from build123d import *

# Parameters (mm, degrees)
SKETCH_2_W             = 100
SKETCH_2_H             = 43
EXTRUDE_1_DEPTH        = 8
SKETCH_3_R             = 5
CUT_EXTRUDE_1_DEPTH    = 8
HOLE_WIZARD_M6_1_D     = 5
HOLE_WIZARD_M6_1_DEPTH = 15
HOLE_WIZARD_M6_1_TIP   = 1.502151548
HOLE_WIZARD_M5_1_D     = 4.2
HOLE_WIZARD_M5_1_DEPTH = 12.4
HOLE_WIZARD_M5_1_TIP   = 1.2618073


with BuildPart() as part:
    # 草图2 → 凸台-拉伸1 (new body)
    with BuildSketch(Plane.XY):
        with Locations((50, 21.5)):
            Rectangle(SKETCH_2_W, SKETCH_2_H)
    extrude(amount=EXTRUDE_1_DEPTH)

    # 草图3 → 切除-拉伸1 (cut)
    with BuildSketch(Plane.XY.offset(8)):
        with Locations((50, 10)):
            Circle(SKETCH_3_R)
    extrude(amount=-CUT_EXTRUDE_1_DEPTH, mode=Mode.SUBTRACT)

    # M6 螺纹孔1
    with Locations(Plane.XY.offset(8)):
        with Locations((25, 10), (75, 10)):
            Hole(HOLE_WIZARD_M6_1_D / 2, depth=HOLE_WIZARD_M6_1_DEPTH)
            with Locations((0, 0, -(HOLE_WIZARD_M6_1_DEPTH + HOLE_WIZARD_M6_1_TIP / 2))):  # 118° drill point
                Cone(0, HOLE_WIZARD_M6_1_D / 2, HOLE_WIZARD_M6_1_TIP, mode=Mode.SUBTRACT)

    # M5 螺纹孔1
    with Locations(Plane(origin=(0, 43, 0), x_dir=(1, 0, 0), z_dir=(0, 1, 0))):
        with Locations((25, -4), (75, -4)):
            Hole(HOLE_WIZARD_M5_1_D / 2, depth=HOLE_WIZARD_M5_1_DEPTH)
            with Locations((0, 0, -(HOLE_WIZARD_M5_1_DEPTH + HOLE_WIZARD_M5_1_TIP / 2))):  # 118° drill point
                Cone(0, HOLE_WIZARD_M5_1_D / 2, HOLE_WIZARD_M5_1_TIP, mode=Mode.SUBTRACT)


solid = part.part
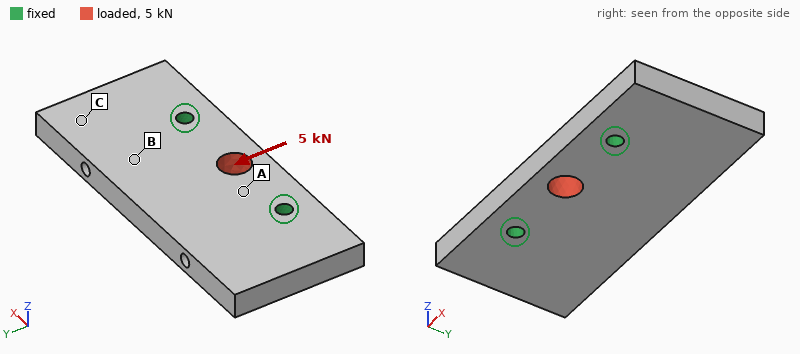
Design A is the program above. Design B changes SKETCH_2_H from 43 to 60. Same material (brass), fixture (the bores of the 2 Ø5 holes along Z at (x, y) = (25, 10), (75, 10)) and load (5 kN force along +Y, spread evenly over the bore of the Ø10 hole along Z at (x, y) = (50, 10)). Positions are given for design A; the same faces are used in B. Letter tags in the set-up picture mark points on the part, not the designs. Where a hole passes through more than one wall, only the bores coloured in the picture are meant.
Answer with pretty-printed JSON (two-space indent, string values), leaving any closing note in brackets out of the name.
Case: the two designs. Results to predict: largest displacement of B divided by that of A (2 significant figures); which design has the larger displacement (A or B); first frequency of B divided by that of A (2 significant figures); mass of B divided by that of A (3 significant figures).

{
  "largest displacement of B divided by that of A": "0.62",
  "which design has the larger displacement": "A",
  "first frequency of B divided by that of A": "0.68",
  "mass of B divided by that of A": "1.40"
}
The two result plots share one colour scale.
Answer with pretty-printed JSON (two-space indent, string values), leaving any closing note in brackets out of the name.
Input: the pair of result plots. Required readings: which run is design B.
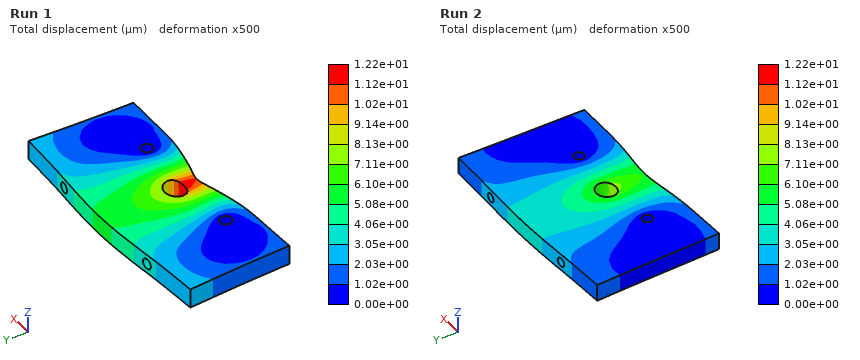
{
  "which run is design B": "Run 2"
}
